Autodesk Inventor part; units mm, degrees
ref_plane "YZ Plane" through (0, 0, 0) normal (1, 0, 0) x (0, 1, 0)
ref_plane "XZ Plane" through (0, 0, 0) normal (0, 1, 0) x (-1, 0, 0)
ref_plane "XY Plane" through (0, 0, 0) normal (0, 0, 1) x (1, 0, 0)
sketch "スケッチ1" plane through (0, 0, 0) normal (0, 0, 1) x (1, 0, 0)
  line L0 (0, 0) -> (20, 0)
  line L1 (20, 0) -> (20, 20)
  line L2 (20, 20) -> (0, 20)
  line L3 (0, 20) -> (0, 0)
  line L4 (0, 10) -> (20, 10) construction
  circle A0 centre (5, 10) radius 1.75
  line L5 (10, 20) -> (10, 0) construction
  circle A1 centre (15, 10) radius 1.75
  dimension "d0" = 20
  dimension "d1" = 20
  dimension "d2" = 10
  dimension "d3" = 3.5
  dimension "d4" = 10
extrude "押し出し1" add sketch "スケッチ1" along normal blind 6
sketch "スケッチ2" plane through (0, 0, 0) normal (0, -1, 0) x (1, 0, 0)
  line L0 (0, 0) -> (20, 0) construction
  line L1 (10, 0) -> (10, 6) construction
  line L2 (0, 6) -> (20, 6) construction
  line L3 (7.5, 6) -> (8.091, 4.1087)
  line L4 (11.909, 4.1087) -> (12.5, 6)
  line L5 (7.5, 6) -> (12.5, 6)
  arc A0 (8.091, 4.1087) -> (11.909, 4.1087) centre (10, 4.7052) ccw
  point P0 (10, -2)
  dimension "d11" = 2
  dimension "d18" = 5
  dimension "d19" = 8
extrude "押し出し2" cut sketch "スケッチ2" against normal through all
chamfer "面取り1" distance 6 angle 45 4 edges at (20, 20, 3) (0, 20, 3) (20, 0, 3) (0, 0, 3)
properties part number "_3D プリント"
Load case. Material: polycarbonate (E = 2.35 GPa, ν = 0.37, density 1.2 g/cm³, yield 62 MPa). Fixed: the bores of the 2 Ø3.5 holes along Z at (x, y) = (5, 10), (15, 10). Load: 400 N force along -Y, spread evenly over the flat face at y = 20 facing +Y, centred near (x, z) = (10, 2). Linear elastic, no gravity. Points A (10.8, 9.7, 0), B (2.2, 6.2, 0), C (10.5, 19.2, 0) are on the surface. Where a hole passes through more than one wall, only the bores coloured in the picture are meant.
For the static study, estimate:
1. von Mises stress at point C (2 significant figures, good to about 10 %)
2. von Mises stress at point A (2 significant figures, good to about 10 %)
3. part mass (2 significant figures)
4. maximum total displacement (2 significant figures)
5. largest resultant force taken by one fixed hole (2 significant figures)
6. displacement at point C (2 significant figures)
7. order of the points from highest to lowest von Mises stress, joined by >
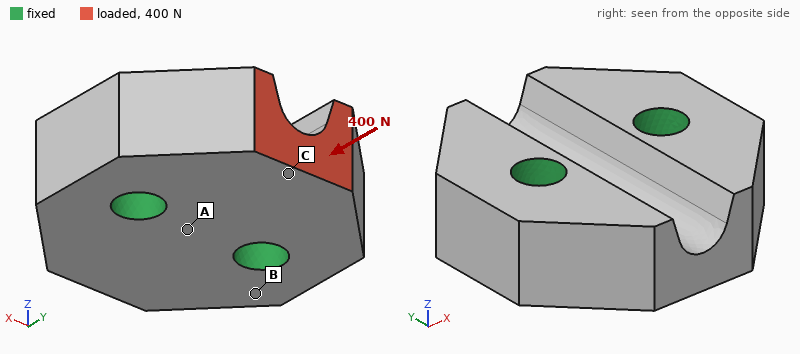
10 MPa
3.3 MPa
1.9 g
47 µm
210 N
42 µm
C > A > B
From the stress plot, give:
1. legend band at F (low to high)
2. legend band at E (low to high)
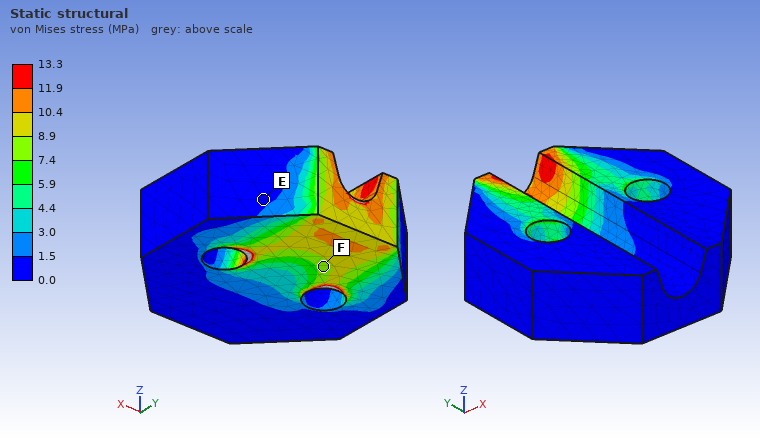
7.4 to 8.9 MPa
0.0 to 1.5 MPa
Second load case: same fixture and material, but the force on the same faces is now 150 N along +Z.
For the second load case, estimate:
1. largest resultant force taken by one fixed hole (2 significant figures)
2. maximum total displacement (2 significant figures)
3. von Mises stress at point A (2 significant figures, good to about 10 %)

75 N
0.13 mm
5.1 MPa
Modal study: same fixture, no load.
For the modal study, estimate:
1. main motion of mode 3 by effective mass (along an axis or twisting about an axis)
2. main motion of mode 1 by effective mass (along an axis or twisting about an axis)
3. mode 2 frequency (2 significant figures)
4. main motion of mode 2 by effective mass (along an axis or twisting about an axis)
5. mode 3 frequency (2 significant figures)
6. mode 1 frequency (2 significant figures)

twisting about Z
twisting about X
16 kHz
along Z
18 kHz
15 kHz
